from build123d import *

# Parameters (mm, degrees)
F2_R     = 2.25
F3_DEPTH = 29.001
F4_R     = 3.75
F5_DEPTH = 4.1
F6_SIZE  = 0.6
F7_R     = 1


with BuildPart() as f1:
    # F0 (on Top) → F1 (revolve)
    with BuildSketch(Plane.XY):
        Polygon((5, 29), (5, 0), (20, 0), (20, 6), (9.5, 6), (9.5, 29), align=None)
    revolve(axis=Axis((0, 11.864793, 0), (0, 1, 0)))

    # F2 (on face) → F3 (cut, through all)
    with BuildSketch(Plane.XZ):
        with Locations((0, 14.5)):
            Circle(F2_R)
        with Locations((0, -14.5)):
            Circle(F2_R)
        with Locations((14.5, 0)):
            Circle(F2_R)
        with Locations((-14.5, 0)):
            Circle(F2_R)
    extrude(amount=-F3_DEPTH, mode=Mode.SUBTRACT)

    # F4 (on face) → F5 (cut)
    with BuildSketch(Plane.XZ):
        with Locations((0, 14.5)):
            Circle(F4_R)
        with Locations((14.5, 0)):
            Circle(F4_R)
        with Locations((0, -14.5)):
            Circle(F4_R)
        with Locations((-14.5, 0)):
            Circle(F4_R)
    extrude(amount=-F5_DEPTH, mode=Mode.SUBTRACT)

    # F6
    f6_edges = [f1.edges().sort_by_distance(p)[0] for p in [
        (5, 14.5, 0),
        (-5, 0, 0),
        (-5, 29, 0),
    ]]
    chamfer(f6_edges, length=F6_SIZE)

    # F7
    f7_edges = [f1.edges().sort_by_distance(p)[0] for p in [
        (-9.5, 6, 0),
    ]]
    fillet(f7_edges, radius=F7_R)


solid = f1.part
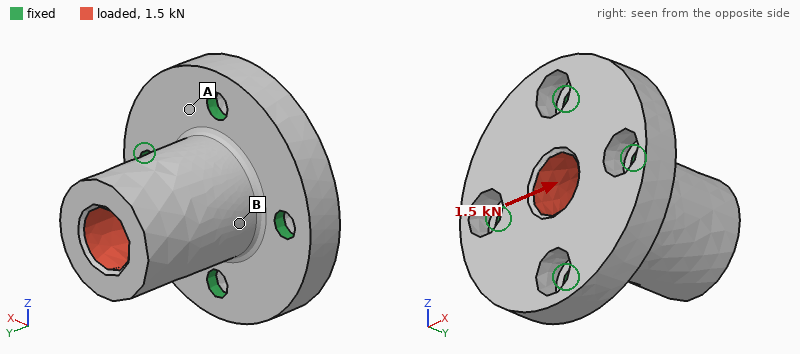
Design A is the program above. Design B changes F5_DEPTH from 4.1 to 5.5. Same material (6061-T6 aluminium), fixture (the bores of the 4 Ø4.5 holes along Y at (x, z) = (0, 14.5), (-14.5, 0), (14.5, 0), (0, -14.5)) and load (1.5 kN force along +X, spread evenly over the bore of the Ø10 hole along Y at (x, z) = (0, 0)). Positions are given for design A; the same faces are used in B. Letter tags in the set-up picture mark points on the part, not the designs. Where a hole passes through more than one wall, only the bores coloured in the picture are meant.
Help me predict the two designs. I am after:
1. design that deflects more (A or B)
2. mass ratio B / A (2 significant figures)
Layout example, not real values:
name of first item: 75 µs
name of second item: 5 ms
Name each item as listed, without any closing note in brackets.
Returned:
design that deflects more: B
mass ratio B / A: 0.99
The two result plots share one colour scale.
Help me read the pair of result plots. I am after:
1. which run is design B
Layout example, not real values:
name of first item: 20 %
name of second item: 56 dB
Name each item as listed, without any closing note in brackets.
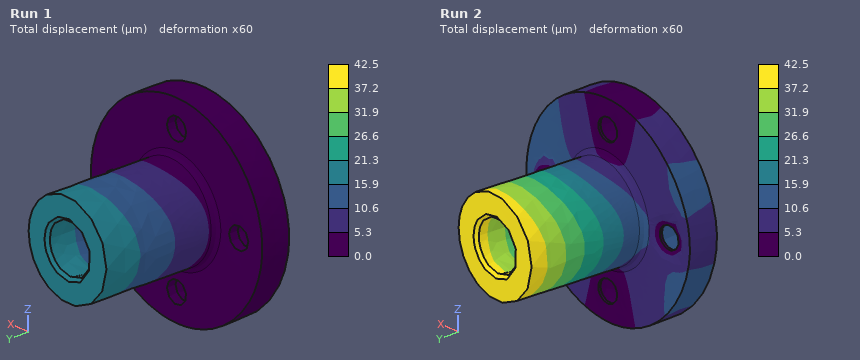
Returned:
which run is design B: Run 2
